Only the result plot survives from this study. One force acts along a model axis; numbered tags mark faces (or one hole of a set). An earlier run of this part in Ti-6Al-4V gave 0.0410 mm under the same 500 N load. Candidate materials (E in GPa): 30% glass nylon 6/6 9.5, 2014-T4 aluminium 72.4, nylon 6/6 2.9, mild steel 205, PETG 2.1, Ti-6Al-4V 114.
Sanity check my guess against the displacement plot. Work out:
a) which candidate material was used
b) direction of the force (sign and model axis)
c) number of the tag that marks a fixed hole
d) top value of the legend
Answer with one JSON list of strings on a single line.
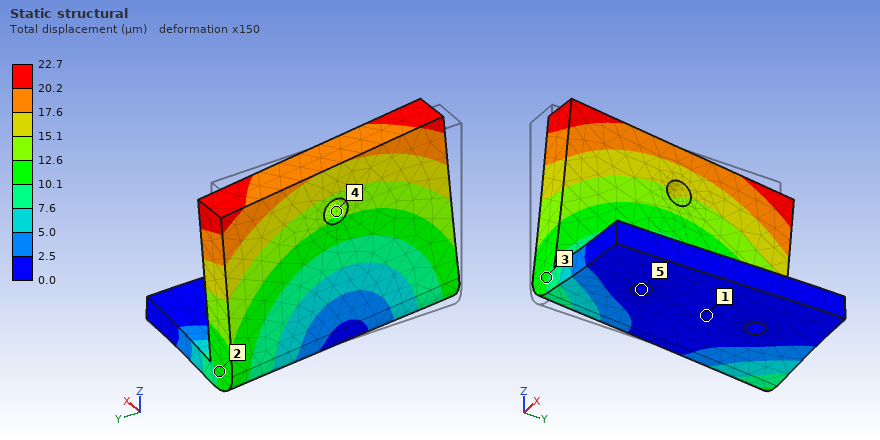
["mild steel", "+Y", "5", "22.7 µm"]
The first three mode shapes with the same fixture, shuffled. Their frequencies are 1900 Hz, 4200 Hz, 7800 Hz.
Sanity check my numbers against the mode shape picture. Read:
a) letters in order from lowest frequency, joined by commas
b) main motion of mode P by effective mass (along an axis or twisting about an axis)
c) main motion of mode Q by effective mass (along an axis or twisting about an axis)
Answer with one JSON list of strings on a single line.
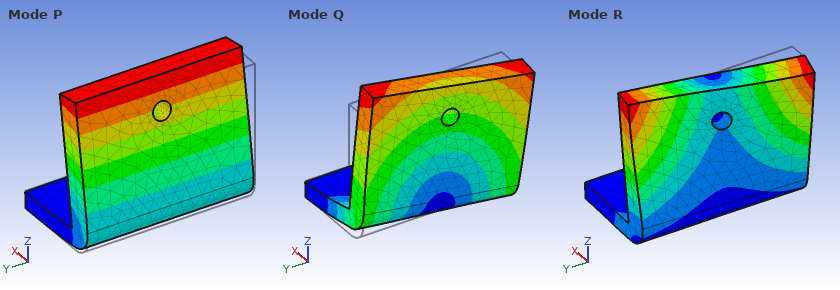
["P, Q, R", "along X", "along Y"]
